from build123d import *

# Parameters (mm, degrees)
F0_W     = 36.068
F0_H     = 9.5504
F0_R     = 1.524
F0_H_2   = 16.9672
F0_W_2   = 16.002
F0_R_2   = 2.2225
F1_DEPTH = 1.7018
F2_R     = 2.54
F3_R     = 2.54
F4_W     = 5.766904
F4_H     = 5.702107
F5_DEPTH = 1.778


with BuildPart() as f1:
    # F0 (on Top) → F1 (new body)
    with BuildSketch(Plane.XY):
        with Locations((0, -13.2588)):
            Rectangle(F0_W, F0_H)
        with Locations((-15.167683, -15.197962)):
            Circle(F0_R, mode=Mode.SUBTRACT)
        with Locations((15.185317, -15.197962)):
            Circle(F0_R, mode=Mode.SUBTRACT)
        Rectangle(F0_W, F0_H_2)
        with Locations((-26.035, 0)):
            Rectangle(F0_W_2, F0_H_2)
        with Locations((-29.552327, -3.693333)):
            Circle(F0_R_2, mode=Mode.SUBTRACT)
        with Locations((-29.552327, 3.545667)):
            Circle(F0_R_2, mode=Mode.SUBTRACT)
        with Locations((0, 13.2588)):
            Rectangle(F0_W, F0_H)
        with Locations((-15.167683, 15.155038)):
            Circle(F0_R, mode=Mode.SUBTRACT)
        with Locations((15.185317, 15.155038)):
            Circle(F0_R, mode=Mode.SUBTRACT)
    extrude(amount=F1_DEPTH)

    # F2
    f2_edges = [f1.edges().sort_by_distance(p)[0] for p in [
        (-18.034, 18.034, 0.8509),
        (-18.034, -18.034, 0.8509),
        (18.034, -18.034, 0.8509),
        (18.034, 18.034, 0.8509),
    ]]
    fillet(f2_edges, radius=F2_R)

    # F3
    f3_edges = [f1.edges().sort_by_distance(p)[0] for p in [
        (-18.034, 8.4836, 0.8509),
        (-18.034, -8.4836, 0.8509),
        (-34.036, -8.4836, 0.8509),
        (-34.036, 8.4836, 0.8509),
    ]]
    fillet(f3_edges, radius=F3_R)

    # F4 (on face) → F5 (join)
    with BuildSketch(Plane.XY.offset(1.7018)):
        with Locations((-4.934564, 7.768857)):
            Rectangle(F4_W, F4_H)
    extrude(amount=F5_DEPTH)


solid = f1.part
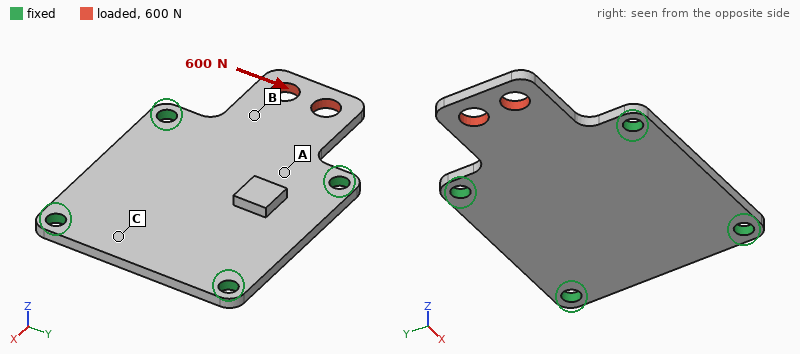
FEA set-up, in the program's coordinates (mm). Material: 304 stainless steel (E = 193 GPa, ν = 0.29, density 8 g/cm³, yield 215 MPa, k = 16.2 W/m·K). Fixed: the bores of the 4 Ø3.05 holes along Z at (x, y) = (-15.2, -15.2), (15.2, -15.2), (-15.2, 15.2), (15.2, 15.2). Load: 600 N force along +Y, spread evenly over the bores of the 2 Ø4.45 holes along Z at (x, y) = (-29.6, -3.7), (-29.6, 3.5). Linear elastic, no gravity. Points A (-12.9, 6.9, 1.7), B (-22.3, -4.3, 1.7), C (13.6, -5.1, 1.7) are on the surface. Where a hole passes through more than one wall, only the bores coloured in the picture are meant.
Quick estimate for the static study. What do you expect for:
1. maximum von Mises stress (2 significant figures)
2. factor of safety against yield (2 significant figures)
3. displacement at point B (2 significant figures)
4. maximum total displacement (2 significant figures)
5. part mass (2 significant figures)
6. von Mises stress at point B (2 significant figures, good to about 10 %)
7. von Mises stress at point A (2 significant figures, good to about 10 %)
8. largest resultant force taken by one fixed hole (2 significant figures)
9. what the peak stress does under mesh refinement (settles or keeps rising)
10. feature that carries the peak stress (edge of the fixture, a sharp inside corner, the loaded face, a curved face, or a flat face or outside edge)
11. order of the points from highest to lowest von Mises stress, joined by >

170 MPa
1.3
4.4 µm
15 µm
21 g
47 MPa
22 MPa
390 N
settles
a curved face
B > A > C
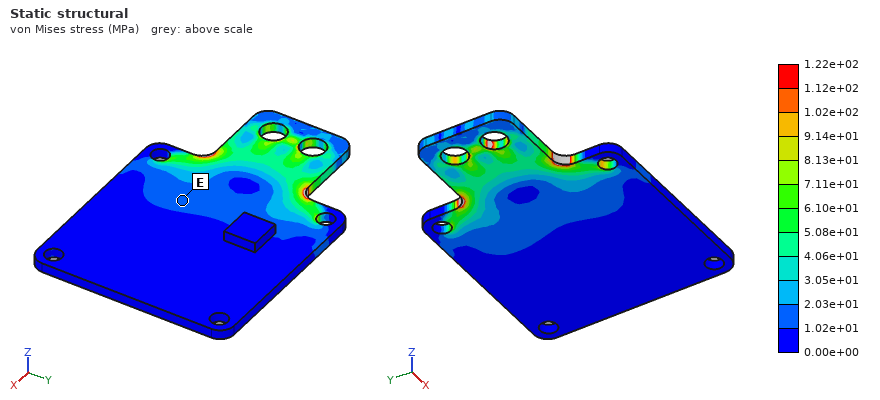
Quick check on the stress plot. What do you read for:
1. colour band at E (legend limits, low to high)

1.02e+01 to 2.03e+01 MPa
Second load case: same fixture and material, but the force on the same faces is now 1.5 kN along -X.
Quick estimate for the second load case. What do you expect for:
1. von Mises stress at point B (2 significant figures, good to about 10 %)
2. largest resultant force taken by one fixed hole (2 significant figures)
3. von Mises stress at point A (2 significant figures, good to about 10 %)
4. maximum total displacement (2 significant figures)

48 MPa
470 N
37 MPa
9.3 µm
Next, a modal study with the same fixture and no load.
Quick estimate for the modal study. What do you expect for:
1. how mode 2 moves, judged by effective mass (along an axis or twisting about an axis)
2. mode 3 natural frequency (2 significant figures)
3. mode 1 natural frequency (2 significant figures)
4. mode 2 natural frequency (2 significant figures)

along Z
9700 Hz
3100 Hz
6600 Hz
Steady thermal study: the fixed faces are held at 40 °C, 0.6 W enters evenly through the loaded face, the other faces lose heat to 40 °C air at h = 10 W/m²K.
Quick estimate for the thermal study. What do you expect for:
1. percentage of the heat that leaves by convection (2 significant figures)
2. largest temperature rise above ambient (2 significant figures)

25 %
25 K
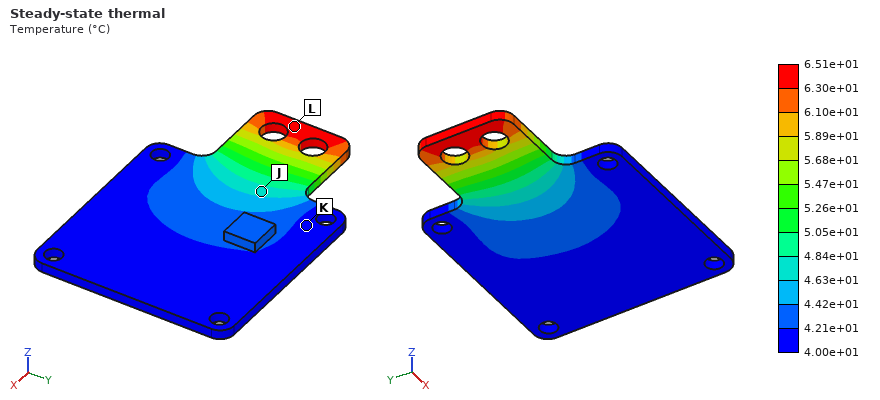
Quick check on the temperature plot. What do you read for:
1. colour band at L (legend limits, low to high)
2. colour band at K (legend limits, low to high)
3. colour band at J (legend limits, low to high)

6.30e+01 to 6.51e+01 °C
4.00e+01 to 4.21e+01 °C
4.63e+01 to 4.84e+01 °C
